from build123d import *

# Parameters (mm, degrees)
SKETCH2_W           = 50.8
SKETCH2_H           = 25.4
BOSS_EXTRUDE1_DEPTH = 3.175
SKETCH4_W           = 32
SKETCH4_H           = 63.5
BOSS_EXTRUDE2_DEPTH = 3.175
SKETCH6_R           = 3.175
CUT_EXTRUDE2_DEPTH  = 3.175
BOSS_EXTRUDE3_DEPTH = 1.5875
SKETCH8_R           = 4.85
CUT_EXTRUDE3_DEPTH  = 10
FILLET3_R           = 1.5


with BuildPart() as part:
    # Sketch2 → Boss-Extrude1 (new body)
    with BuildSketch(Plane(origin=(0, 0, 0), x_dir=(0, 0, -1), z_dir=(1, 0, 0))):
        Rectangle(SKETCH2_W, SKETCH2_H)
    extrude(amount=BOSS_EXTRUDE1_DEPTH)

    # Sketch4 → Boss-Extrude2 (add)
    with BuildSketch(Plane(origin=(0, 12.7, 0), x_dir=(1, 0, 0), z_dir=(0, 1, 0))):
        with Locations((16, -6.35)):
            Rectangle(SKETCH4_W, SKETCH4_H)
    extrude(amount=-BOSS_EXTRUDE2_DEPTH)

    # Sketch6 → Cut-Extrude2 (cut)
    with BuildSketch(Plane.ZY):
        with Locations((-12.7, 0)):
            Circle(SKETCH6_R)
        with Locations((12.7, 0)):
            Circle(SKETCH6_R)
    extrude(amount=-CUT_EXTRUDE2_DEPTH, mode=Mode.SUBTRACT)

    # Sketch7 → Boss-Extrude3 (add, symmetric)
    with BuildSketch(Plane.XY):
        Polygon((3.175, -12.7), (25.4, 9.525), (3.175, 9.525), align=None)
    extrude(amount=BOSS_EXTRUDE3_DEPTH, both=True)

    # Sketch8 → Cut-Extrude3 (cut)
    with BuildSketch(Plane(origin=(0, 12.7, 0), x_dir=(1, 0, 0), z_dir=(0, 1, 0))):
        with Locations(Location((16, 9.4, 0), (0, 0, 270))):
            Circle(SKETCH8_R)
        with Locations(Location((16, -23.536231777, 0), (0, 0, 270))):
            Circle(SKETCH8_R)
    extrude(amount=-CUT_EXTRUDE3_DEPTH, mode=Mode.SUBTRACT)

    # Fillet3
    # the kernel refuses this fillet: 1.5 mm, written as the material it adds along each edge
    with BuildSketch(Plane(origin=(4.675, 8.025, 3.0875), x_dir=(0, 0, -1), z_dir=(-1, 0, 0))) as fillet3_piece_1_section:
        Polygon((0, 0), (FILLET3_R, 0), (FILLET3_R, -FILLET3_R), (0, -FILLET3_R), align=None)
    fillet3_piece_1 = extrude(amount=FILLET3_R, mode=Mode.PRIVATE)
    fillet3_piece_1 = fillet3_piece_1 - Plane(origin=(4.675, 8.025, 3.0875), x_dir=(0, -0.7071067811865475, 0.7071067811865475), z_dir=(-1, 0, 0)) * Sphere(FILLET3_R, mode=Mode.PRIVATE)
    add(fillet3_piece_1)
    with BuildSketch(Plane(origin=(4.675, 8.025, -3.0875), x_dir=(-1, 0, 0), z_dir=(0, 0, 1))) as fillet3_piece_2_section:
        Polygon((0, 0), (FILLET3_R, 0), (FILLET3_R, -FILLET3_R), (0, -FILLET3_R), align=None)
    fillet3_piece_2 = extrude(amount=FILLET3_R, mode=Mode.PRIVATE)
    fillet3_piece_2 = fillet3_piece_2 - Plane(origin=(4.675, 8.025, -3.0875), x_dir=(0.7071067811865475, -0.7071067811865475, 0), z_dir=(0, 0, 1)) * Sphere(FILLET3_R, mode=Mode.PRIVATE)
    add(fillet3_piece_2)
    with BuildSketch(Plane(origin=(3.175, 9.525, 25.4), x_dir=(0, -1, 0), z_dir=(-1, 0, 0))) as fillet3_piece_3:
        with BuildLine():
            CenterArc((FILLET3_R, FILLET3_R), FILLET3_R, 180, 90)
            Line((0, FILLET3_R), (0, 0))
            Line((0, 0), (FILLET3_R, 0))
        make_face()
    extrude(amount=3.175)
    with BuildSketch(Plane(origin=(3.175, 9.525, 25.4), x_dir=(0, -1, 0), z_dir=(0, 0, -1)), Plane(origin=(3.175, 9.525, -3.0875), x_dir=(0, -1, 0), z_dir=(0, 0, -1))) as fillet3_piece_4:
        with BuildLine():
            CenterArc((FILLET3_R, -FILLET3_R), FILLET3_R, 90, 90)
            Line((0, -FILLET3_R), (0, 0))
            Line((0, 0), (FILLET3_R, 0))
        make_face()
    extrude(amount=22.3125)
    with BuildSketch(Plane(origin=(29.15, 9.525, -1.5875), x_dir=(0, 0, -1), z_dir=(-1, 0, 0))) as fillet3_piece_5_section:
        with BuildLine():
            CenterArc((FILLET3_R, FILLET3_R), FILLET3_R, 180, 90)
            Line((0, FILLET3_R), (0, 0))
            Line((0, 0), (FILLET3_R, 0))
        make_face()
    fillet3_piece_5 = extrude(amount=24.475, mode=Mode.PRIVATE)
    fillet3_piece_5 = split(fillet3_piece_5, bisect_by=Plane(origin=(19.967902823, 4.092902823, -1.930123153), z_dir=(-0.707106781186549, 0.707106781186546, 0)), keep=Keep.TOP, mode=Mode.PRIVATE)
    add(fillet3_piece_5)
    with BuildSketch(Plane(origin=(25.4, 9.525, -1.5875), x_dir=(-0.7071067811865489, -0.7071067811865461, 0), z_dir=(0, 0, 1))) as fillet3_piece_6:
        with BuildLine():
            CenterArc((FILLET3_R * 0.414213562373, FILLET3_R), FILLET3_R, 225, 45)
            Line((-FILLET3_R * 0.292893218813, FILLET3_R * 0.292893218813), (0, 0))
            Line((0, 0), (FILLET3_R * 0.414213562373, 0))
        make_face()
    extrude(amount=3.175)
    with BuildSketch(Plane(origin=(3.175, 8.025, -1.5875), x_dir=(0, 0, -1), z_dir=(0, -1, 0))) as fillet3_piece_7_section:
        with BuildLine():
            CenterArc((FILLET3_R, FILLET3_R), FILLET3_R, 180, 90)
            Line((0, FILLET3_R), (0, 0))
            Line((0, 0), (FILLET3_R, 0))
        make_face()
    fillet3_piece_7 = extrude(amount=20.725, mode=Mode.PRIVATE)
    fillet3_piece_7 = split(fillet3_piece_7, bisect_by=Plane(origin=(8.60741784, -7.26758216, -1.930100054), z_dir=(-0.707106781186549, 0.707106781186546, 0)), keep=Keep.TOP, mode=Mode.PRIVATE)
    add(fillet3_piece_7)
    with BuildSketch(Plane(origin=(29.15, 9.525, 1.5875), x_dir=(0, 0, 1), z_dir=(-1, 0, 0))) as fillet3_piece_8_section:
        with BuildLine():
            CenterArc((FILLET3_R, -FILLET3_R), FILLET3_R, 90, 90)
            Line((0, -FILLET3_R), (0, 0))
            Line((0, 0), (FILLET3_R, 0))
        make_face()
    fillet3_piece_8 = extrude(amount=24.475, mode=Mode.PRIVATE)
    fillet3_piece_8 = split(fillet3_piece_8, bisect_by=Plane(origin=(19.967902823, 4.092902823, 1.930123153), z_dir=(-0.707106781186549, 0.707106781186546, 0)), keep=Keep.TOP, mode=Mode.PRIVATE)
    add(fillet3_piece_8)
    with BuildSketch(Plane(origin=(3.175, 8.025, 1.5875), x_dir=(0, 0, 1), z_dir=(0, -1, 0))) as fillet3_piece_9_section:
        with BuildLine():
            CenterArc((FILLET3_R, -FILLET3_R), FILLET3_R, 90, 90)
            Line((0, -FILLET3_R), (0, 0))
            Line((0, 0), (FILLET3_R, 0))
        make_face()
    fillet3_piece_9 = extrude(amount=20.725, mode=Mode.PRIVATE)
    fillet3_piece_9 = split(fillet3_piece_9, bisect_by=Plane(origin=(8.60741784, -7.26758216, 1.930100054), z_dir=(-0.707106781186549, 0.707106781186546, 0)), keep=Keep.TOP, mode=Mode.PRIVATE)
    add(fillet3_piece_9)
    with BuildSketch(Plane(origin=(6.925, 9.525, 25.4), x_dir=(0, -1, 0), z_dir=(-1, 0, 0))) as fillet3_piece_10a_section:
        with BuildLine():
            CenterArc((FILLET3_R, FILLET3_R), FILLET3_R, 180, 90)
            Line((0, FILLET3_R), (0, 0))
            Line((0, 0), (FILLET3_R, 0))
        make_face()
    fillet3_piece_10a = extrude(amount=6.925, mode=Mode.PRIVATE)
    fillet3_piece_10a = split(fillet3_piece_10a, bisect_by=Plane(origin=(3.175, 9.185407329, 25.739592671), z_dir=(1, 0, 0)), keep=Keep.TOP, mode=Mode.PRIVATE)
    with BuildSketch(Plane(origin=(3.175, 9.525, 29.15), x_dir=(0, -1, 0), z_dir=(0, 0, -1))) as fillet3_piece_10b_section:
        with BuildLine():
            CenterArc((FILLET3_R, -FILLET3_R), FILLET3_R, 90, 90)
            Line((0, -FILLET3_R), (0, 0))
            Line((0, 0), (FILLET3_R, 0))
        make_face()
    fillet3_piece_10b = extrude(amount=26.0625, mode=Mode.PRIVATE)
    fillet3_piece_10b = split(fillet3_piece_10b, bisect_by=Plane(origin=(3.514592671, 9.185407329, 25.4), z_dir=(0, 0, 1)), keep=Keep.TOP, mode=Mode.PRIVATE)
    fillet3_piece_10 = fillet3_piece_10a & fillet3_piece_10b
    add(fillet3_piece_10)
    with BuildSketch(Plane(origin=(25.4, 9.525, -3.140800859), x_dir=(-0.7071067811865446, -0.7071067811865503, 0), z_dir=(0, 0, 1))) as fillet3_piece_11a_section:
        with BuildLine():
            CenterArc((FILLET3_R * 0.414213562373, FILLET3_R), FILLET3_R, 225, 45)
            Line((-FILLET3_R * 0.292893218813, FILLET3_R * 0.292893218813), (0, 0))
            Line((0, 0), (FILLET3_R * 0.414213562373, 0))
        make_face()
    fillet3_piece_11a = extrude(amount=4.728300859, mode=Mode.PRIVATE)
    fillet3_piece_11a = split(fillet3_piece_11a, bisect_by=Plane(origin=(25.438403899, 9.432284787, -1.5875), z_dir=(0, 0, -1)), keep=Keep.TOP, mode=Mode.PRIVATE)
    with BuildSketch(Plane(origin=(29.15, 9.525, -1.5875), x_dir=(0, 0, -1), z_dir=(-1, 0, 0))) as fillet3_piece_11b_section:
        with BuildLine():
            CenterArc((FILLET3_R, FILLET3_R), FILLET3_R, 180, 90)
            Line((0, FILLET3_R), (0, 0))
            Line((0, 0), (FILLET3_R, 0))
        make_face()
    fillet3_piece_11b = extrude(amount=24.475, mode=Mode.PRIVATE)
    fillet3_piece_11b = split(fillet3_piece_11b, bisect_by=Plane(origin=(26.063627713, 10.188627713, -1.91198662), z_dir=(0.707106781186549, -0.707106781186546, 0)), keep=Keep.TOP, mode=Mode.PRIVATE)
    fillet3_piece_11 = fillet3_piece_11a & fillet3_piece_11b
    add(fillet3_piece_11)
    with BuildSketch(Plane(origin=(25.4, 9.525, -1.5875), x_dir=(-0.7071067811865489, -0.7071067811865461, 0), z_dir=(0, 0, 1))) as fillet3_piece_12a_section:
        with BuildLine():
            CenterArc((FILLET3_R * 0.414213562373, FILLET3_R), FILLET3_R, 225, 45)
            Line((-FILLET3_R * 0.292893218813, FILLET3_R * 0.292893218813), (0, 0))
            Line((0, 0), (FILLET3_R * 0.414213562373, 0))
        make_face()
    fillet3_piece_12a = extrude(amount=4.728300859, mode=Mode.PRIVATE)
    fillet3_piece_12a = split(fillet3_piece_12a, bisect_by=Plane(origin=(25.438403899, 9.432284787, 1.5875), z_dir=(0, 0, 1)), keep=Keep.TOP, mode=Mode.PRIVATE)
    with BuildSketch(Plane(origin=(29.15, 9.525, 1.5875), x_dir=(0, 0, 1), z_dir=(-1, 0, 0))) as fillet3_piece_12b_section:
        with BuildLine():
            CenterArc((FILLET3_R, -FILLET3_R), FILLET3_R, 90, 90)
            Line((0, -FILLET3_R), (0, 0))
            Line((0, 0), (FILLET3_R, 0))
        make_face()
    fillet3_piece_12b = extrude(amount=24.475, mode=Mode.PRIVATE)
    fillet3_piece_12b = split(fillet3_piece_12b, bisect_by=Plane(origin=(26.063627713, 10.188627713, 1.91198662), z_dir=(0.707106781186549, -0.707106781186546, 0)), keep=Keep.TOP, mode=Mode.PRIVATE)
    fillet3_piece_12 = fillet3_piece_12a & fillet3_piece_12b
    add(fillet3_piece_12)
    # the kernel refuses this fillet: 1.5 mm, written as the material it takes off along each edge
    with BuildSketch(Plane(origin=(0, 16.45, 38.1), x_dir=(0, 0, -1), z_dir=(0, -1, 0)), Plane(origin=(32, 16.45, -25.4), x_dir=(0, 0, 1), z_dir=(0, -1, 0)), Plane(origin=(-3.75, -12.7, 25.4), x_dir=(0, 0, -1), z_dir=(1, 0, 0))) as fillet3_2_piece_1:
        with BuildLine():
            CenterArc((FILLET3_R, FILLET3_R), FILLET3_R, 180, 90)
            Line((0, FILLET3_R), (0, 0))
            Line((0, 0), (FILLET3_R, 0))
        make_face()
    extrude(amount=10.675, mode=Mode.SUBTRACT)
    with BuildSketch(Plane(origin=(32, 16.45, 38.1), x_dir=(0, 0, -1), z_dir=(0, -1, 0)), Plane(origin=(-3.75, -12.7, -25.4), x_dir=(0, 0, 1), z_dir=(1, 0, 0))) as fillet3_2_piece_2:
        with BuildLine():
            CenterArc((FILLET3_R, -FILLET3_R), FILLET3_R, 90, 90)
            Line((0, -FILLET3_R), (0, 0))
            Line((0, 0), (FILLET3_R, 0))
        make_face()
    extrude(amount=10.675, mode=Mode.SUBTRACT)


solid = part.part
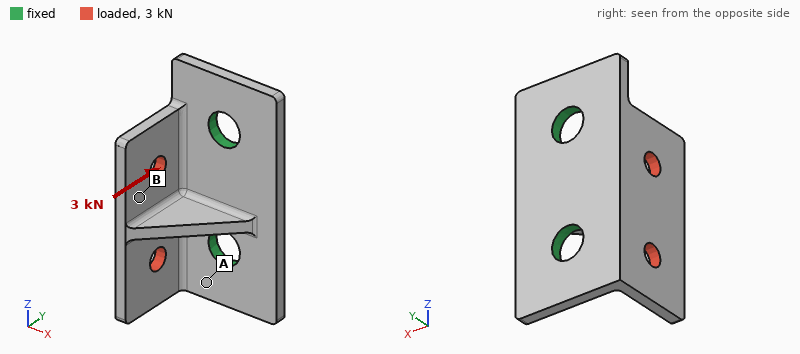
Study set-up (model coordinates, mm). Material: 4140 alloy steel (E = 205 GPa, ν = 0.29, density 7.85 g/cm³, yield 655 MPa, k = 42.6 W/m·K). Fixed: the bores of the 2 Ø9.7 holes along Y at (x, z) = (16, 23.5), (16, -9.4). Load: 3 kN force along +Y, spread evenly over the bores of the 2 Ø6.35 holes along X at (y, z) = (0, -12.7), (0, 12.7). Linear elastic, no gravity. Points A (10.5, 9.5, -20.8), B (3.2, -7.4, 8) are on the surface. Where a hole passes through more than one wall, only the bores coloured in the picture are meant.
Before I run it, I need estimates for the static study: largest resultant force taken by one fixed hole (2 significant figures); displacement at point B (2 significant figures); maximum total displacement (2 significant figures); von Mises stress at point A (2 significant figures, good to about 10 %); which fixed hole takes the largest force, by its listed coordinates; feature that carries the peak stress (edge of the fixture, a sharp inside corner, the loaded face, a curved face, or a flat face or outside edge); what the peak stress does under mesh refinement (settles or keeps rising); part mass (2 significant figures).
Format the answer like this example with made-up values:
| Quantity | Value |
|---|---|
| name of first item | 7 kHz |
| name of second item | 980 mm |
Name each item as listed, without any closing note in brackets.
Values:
| Quantity | Value |
|---|---|
| largest resultant force taken by one fixed hole | 2.2 kN |
| displacement at point B | 55 µm |
| maximum total displacement | 88 µm |
| von Mises stress at point A | 100 MPa |
| which fixed hole takes the largest force, by its listed coordinates | (16, -9.4) |
| feature that carries the peak stress | edge of the fixture |
| what the peak stress does under mesh refinement | keeps rising |
| part mass | 80 g |
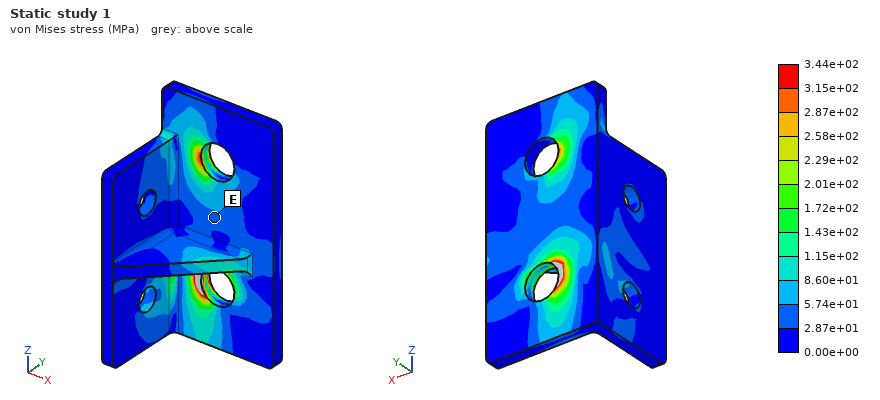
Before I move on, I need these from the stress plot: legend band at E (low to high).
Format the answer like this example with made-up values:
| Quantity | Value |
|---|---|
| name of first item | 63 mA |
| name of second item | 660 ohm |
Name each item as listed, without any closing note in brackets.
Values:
| Quantity | Value |
|---|---|
| legend band at E | 2.87e+01 to 5.74e+01 MPa |
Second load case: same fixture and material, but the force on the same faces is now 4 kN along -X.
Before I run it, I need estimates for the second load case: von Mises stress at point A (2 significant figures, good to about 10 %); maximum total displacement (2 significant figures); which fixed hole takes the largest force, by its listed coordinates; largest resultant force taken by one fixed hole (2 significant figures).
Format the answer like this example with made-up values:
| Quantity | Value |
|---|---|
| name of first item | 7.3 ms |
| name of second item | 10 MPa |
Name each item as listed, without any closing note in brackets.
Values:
| Quantity | Value |
|---|---|
| von Mises stress at point A | 160 MPa |
| maximum total displacement | 0.17 mm |
| which fixed hole takes the largest force, by its listed coordinates | (16, -9.4) |
| largest resultant force taken by one fixed hole | 2.9 kN |
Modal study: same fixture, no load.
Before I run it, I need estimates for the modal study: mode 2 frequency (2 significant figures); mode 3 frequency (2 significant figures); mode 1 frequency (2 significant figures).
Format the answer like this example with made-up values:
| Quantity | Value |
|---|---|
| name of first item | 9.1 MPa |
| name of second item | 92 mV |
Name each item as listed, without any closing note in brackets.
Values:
| Quantity | Value |
|---|---|
| mode 2 frequency | 5800 Hz |
| mode 3 frequency | 8300 Hz |
| mode 1 frequency | 4800 Hz |
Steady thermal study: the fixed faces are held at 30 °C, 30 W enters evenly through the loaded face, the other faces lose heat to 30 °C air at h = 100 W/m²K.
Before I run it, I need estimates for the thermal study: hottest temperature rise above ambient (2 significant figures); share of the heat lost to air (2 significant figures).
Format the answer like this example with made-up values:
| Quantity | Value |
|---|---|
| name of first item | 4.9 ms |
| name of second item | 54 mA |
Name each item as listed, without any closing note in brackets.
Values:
| Quantity | Value |
|---|---|
| hottest temperature rise above ambient | 64 K |
| share of the heat lost to air | 48 % |
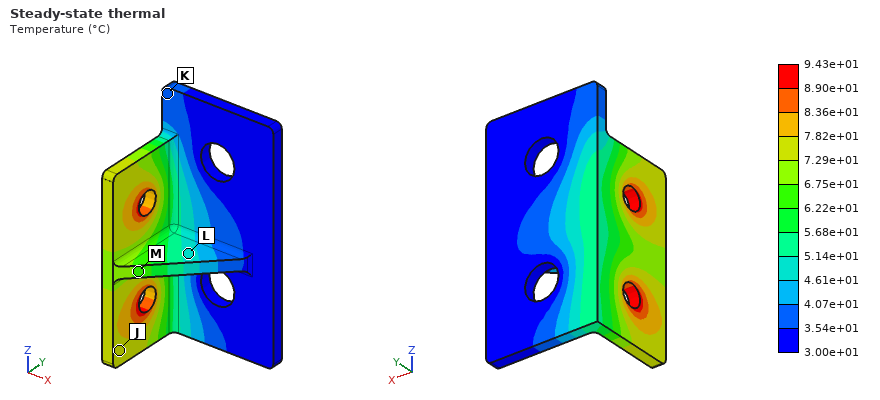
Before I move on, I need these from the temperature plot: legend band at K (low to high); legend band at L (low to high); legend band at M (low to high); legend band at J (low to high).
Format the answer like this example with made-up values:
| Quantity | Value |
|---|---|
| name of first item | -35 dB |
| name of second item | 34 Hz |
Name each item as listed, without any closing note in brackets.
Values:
| Quantity | Value |
|---|---|
| legend band at K | 3.54e+01 to 4.07e+01 °C |
| legend band at L | 4.61e+01 to 5.14e+01 °C |
| legend band at M | 6.22e+01 to 6.75e+01 °C |
| legend band at J | 7.29e+01 to 7.82e+01 °C |
